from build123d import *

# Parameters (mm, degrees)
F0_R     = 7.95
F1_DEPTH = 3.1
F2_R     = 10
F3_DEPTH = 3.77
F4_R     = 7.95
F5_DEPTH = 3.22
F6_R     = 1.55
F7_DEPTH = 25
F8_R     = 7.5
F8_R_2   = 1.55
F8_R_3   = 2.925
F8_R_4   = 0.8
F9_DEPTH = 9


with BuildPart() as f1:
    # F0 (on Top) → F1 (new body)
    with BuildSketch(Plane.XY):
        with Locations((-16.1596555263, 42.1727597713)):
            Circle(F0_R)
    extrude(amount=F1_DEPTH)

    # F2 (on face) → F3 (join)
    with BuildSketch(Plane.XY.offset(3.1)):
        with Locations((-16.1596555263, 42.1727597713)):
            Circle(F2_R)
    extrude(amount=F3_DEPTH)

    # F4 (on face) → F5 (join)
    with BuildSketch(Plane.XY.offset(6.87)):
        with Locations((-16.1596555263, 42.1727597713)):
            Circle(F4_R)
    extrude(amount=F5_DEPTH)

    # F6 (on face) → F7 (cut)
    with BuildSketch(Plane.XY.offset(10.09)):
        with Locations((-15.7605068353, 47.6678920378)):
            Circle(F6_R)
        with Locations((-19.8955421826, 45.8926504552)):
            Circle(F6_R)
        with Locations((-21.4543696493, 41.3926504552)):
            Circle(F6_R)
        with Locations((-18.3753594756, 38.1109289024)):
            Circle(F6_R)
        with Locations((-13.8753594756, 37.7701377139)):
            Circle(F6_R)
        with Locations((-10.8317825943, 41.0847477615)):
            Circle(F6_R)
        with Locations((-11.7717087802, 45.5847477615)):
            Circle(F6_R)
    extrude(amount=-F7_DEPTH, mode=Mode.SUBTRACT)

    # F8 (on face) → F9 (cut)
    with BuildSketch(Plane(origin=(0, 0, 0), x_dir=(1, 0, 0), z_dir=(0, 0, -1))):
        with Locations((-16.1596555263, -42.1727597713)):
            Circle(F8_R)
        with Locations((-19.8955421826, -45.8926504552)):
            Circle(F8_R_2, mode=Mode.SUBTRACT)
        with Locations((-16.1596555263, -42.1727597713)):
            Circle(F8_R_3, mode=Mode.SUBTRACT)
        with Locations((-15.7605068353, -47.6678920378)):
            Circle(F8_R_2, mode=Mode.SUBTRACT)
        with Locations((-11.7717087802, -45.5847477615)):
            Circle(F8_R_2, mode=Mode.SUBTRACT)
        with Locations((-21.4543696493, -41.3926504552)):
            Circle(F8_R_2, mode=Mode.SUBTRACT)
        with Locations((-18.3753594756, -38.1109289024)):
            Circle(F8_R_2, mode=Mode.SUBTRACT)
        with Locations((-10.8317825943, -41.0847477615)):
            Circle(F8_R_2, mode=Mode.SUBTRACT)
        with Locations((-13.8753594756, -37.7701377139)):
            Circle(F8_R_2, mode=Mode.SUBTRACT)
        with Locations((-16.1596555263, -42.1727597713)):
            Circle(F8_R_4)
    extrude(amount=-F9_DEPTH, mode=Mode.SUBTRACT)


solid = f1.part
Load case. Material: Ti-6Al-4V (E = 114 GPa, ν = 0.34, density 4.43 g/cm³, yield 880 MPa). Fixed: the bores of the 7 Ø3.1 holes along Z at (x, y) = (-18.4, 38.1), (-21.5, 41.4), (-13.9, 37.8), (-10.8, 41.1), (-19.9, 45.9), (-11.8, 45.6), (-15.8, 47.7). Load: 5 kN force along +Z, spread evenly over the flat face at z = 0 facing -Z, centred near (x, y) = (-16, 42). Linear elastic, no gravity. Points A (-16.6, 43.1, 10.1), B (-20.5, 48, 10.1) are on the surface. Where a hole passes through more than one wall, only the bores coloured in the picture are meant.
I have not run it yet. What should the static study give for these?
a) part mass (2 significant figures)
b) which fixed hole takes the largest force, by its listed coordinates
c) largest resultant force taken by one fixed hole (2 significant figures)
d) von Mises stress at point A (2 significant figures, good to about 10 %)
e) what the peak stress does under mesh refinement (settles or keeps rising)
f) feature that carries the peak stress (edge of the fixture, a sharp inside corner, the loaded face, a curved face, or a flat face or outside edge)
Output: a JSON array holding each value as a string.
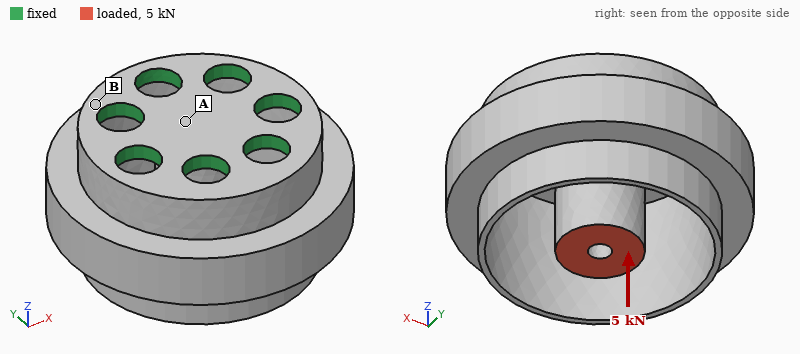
["4.5 g", "(-18.4, 38.1)", "1.2 kN", "180 MPa", "keeps rising", "edge of the fixture"]
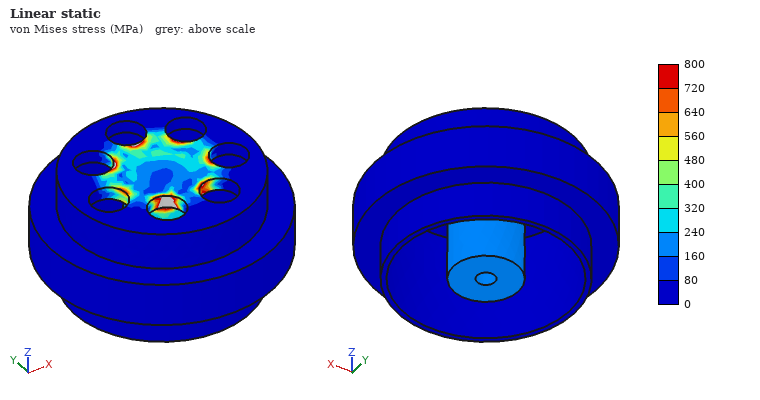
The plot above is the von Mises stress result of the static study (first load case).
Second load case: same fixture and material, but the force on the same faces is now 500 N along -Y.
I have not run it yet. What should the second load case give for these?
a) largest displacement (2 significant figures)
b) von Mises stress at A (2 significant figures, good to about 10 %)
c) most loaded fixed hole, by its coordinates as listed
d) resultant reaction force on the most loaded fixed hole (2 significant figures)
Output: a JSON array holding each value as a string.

["44 µm", "73 MPa", "(-18.4, 38.1)", "530 N"]
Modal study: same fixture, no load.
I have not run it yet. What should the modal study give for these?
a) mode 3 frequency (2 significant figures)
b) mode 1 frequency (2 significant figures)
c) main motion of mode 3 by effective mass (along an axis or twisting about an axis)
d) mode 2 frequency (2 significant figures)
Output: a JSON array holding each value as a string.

["28 kHz", "25 kHz", "along Y", "26 kHz"]
